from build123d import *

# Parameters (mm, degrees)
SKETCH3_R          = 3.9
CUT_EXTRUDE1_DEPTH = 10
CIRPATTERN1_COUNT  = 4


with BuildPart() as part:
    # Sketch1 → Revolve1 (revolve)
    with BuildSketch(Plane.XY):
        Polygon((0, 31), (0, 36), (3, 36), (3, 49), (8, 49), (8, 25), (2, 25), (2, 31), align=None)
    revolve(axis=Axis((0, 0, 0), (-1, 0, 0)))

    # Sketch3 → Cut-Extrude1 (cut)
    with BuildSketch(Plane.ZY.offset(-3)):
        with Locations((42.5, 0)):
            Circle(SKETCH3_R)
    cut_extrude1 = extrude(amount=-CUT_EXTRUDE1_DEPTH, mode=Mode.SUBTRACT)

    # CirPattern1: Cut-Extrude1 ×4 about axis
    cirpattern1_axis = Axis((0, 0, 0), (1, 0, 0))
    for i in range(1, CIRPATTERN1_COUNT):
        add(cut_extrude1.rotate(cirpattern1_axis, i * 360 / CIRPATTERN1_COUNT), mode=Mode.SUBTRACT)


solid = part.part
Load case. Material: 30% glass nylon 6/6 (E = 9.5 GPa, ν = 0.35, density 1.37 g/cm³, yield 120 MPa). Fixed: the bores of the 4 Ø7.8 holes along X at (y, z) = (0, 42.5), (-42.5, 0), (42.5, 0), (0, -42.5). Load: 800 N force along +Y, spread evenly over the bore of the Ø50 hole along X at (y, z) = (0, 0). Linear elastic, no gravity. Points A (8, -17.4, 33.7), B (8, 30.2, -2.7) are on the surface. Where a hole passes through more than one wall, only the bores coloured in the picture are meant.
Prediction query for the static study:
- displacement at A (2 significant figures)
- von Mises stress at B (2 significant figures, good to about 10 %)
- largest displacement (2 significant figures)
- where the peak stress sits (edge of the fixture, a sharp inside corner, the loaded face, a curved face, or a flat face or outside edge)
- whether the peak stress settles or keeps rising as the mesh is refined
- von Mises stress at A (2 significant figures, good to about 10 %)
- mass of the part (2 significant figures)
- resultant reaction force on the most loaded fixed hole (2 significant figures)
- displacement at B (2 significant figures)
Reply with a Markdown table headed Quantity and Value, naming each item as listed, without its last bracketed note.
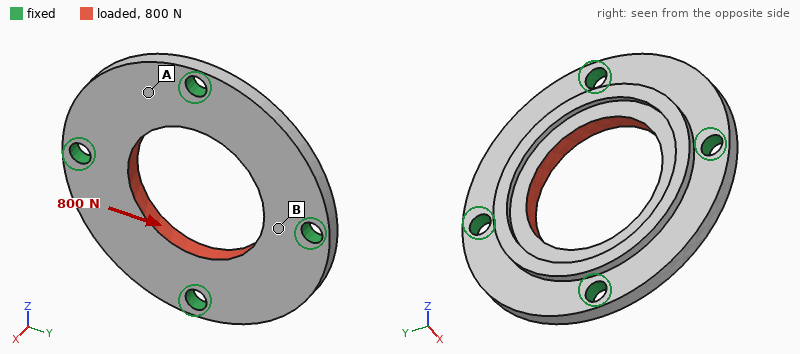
| Quantity | Value |
|---|---|
| displacement at A | 4.1 µm |
| von Mises stress at B | 1.8 MPa |
| largest displacement | 6.2 µm |
| where the peak stress sits | edge of the fixture |
| whether the peak stress settles or keeps rising as the mesh is refined | keeps rising |
| von Mises stress at A | 0.87 MPa |
| mass of the part | 43 g |
| resultant reaction force on the most loaded fixed hole | 200 N |
| displacement at B | 1.9 µm |
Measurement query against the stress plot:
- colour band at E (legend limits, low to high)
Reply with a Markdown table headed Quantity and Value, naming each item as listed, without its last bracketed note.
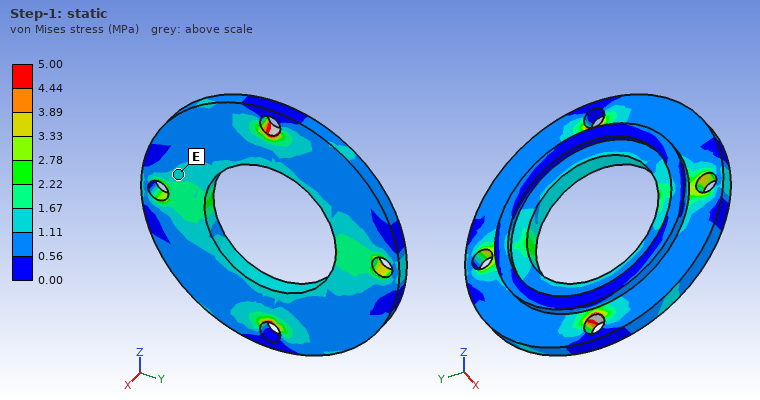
| Quantity | Value |
|---|---|
| colour band at E | 1.11 to 1.67 MPa |
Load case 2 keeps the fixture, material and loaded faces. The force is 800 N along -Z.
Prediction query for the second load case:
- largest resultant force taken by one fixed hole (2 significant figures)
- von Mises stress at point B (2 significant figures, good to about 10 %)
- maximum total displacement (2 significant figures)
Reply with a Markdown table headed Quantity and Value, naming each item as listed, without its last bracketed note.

| Quantity | Value |
|---|---|
| largest resultant force taken by one fixed hole | 200 N |
| von Mises stress at point B | 1.0 MPa |
| maximum total displacement | 6.2 µm |
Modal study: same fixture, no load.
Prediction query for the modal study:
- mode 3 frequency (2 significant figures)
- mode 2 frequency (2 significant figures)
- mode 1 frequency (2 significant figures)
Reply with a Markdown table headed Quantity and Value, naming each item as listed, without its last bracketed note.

| Quantity | Value |
|---|---|
| mode 3 frequency | 3900 Hz |
| mode 2 frequency | 3900 Hz |
| mode 1 frequency | 3600 Hz |
